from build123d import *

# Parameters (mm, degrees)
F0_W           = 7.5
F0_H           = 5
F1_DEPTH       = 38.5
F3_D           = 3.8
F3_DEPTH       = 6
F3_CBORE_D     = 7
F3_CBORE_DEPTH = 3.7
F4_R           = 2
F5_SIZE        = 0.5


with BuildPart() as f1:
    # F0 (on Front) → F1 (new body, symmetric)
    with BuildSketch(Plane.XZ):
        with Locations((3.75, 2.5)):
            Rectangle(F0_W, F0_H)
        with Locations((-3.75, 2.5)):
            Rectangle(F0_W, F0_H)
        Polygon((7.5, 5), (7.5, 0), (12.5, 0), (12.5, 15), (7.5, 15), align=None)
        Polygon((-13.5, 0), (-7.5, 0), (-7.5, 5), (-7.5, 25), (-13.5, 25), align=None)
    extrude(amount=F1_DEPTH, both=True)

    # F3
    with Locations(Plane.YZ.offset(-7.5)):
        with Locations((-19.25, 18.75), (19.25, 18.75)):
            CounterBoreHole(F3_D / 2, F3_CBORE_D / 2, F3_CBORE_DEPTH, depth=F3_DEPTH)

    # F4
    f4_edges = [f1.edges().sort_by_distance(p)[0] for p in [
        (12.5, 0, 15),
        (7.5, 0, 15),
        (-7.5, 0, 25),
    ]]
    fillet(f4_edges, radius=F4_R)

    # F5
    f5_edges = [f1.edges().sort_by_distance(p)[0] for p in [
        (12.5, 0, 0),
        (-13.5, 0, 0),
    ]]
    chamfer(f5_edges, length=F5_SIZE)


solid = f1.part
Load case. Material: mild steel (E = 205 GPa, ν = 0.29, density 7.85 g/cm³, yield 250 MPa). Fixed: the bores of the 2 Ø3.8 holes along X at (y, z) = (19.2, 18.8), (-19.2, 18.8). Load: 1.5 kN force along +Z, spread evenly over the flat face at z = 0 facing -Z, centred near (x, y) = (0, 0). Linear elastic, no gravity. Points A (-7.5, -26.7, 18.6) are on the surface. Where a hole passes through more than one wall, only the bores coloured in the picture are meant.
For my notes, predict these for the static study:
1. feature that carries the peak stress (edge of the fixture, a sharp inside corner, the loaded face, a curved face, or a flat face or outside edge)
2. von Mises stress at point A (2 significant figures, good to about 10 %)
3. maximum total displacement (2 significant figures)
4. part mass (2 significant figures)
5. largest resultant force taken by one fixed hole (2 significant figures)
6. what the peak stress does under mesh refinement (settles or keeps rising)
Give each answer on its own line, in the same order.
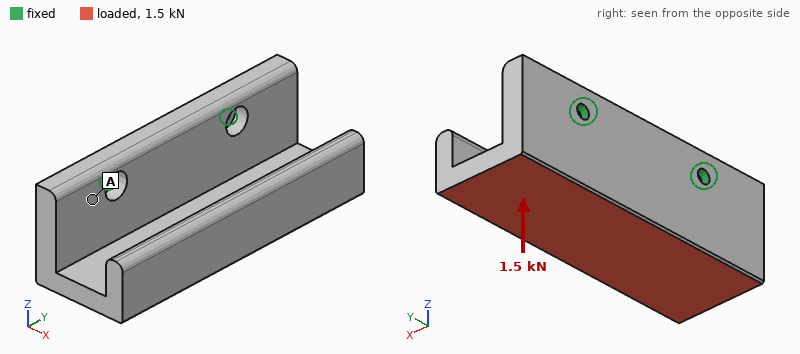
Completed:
edge of the fixture
51 MPa
100 µm
180 g
750 N
keeps rising
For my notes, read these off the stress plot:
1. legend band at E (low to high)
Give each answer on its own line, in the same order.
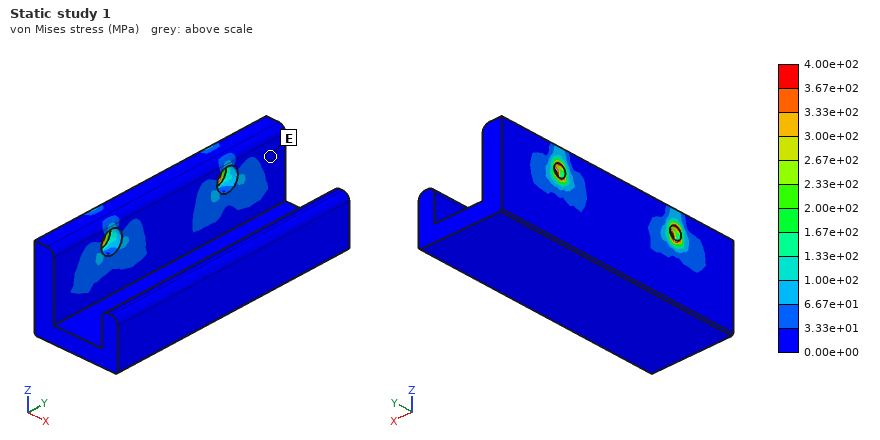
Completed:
0.00e+00 to 3.33e+01 MPa
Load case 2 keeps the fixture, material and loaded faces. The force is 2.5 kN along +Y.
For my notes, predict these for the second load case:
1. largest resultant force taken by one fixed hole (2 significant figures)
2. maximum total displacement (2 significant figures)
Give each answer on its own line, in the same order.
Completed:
1.9 kN
24 µm
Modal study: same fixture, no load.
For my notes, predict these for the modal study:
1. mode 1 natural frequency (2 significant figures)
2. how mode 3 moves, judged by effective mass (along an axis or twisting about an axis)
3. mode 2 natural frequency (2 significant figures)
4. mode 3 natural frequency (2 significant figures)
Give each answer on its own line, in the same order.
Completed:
1700 Hz
along X
3100 Hz
5500 Hz
